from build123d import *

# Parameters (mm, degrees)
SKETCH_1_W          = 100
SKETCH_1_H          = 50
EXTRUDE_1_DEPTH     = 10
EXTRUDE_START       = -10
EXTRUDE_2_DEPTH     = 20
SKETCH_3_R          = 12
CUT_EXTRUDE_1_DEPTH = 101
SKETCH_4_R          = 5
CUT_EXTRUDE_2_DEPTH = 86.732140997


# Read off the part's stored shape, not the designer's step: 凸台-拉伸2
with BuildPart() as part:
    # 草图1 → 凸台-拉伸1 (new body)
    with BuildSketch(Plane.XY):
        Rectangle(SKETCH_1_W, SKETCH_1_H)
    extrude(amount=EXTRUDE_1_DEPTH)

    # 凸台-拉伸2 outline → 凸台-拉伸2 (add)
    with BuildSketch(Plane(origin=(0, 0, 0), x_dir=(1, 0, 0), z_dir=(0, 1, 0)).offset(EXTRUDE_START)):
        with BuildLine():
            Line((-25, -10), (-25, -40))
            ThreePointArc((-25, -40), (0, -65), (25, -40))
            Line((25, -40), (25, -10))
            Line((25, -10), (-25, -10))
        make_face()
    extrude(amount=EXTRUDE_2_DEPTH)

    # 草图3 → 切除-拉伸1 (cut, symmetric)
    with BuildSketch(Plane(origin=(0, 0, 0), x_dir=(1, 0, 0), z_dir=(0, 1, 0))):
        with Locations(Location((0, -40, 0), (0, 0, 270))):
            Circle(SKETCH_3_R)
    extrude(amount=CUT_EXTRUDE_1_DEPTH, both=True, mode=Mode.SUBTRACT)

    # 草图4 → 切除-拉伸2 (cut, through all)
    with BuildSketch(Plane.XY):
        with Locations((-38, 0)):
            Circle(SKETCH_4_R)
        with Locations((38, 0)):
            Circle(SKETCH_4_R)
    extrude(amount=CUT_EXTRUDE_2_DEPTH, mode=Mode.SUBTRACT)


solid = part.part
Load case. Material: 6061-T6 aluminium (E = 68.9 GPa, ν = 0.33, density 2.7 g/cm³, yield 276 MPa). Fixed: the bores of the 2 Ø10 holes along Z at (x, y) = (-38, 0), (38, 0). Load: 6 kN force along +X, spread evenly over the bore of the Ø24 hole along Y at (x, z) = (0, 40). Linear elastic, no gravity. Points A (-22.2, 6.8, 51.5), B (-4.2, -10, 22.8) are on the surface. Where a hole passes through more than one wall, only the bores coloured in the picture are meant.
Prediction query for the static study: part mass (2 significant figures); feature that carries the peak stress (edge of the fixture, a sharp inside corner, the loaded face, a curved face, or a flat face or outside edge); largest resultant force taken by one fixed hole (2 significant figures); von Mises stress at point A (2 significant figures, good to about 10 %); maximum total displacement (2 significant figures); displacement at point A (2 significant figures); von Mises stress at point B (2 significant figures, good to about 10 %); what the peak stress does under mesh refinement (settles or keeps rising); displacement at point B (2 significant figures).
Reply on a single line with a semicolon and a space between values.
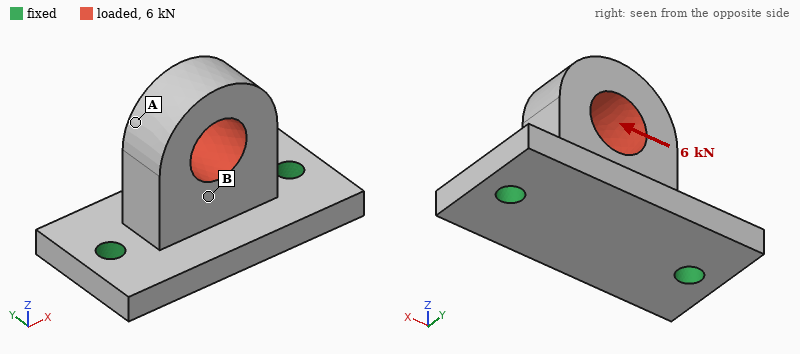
240 g; edge of the fixture; 4.6 kN; 10 MPa; 57 µm; 51 µm; 22 MPa; keeps rising; 15 µm
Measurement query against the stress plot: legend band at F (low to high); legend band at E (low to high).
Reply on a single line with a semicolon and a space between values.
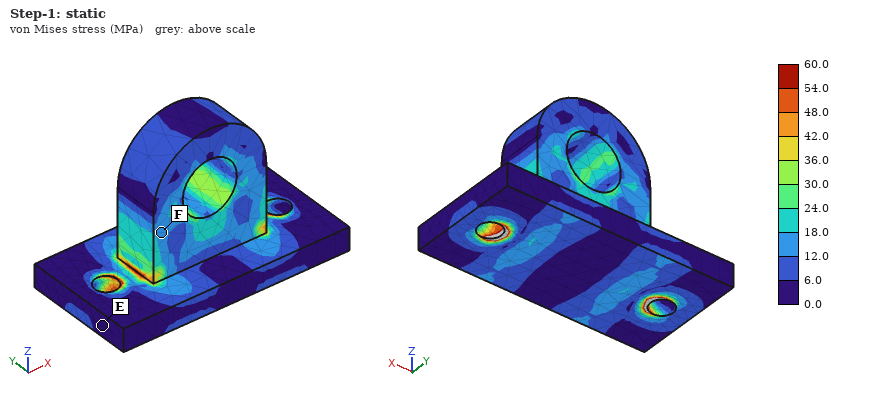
12.0 to 18.0 MPa; 0.0 to 6.0 MPa
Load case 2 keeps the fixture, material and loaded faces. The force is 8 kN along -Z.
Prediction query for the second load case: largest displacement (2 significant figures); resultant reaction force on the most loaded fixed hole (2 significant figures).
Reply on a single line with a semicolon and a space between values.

27 µm; 4.2 kN
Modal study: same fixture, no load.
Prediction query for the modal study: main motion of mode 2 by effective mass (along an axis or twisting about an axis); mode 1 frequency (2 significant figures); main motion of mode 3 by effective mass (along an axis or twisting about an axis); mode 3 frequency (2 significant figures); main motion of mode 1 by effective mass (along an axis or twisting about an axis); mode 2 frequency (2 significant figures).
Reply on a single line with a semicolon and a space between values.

along X; 2600 Hz; along Z; 7200 Hz; along Y; 6200 Hz
